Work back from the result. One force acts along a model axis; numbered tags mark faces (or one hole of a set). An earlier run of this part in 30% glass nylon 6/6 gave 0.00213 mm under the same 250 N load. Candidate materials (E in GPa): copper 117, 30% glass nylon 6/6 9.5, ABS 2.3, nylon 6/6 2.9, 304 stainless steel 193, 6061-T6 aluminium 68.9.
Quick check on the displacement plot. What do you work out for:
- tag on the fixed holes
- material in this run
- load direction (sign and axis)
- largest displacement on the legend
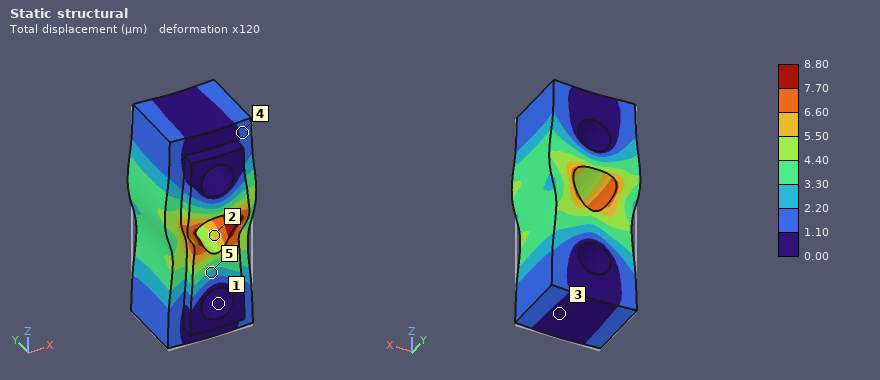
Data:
1
ABS
+Z
8.80 µm
